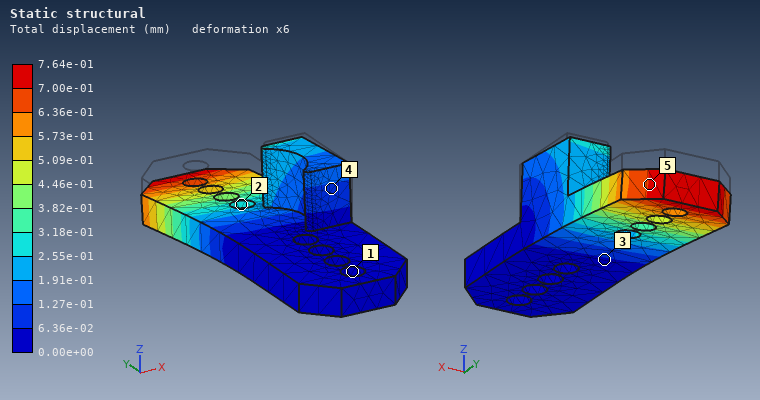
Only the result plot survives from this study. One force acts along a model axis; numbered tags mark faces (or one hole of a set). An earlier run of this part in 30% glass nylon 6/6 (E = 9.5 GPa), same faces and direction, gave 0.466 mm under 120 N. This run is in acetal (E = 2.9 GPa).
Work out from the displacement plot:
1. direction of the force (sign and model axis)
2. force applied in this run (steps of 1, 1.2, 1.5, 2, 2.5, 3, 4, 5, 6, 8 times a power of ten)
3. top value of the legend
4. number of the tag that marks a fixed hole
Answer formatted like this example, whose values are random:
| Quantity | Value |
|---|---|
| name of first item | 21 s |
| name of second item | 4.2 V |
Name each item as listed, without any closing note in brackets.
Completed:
| Quantity | Value |
|---|---|
| direction of the force | -Z |
| force applied in this run | 60 N |
| top value of the legend | 7.64e-01 mm |
| number of the tag that marks a fixed hole | 1 |
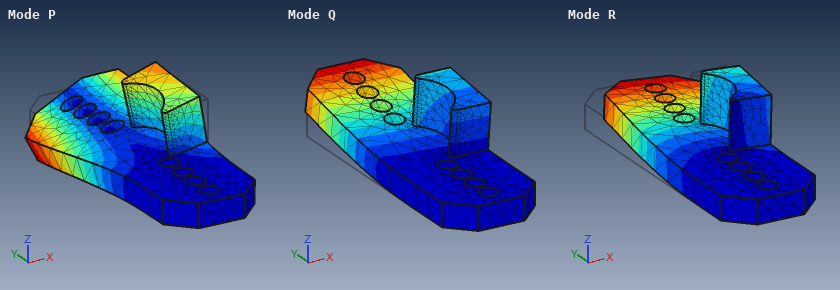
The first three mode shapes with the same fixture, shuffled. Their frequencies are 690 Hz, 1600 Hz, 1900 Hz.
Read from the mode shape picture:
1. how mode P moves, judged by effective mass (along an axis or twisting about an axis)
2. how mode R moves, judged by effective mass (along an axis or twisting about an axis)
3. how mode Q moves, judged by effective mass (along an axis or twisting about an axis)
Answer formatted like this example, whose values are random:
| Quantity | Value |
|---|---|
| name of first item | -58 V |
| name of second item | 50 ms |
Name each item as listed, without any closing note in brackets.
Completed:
| Quantity | Value |
|---|---|
| how mode P moves, judged by effective mass | twisting about Y |
| how mode R moves, judged by effective mass | along X |
| how mode Q moves, judged by effective mass | along Z |
